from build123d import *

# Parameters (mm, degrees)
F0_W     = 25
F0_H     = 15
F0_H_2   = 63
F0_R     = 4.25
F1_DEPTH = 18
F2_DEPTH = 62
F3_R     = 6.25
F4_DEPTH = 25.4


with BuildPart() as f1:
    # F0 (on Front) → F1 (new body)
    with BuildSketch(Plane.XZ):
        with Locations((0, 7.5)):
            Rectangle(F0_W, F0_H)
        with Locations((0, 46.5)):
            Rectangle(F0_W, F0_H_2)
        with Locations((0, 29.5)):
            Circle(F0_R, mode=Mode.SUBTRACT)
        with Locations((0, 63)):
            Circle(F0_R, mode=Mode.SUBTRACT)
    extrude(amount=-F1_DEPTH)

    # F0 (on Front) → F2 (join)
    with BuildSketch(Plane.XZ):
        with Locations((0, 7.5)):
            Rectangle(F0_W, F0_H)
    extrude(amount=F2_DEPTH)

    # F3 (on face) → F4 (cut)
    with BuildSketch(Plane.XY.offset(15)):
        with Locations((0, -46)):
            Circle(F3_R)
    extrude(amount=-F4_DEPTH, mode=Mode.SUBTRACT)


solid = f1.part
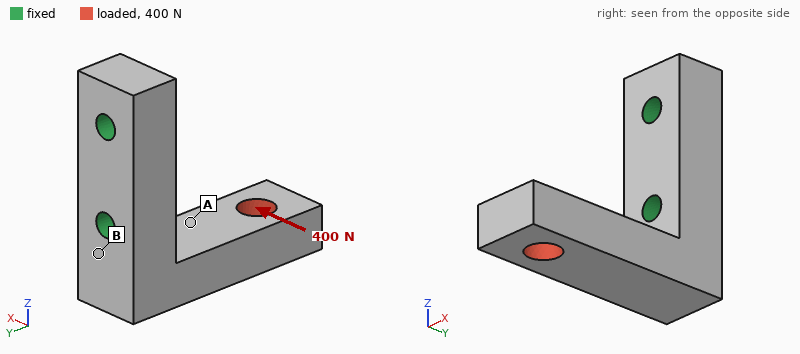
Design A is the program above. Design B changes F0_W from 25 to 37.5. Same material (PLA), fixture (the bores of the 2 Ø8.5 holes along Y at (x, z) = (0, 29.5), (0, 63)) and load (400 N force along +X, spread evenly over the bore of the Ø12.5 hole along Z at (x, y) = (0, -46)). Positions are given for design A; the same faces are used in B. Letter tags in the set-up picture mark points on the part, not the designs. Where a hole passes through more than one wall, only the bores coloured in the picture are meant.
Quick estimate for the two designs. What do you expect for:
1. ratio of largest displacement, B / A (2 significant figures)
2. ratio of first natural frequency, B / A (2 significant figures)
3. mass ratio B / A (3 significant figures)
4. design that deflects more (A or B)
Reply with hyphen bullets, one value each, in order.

- 0.50
- 0.96
- 1.54
- A
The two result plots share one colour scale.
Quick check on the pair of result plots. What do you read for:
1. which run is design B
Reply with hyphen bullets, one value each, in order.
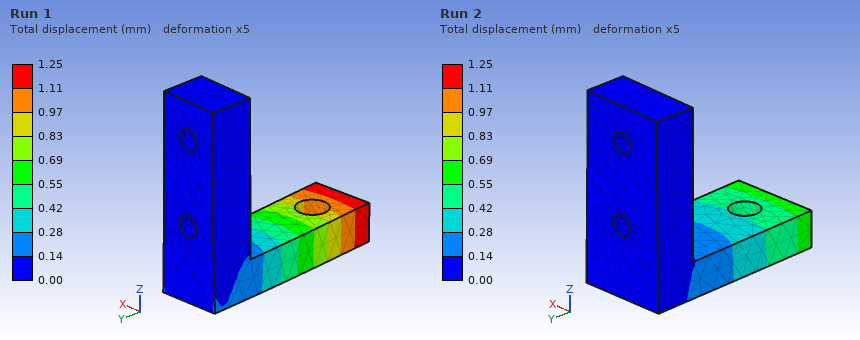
- Run 2
